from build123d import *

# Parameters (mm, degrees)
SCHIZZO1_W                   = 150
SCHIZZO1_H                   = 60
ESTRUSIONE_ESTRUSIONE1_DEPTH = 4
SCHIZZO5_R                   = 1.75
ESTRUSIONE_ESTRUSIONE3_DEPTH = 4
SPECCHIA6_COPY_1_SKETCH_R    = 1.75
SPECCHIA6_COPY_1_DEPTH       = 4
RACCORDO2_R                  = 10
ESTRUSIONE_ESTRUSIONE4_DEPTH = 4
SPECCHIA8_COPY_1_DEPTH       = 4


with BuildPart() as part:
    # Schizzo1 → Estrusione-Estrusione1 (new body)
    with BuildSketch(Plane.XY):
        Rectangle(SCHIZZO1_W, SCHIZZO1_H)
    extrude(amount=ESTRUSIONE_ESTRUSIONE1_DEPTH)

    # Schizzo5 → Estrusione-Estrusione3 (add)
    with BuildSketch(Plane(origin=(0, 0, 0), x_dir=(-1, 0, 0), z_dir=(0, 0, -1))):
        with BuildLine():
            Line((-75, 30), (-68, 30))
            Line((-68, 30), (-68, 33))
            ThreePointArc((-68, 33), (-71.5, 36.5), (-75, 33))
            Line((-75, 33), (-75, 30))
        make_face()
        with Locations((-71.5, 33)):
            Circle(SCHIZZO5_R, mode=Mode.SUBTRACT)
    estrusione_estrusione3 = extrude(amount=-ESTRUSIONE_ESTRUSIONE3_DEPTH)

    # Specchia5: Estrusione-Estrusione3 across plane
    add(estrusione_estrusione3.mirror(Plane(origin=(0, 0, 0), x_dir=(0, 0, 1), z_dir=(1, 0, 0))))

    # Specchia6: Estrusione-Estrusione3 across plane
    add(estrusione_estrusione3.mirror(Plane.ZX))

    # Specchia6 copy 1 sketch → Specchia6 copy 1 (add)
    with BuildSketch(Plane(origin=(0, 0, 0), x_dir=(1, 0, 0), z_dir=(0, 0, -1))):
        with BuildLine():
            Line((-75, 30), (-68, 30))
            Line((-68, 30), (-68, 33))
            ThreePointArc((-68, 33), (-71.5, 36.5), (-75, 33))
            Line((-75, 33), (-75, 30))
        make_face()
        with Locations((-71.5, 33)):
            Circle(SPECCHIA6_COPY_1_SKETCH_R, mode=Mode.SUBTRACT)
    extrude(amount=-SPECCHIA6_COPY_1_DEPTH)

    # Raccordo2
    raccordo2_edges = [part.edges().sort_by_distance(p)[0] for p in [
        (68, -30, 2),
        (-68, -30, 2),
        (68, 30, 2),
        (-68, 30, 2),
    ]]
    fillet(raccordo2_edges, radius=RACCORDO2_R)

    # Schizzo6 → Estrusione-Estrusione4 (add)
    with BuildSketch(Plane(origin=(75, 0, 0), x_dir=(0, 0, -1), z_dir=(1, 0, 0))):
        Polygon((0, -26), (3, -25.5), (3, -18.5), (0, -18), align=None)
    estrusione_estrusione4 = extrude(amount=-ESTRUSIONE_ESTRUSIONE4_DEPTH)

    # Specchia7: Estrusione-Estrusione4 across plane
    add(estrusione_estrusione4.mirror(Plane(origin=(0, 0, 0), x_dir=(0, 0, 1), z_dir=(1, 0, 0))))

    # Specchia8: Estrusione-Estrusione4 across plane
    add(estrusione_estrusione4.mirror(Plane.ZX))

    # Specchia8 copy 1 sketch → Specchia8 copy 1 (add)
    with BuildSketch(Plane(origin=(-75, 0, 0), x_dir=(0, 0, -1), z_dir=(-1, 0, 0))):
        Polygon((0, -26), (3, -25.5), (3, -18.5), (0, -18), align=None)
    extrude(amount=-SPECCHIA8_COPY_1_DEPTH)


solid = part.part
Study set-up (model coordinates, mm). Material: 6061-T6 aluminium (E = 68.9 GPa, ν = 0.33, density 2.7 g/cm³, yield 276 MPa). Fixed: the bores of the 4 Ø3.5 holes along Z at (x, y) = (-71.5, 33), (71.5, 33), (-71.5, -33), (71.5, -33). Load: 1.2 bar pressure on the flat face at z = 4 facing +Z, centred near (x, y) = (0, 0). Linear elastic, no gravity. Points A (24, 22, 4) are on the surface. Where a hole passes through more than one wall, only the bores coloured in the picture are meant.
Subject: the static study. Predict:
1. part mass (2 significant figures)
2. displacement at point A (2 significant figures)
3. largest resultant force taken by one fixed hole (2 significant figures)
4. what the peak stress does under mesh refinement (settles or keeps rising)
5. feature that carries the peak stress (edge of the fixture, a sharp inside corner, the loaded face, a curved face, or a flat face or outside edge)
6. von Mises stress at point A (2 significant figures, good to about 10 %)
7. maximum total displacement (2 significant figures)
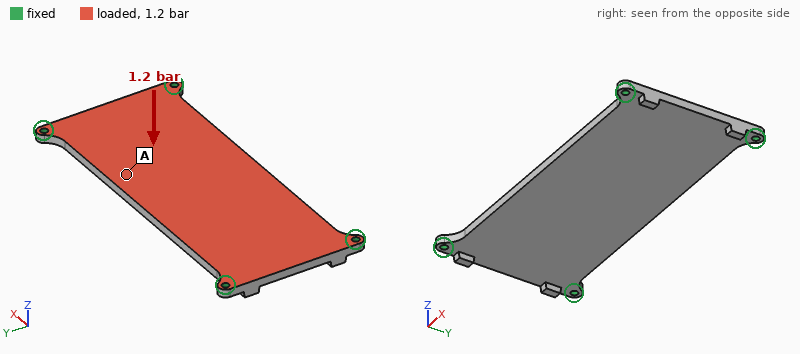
100 g
0.51 mm
280 N
keeps rising
edge of the fixture
41 MPa
0.63 mm
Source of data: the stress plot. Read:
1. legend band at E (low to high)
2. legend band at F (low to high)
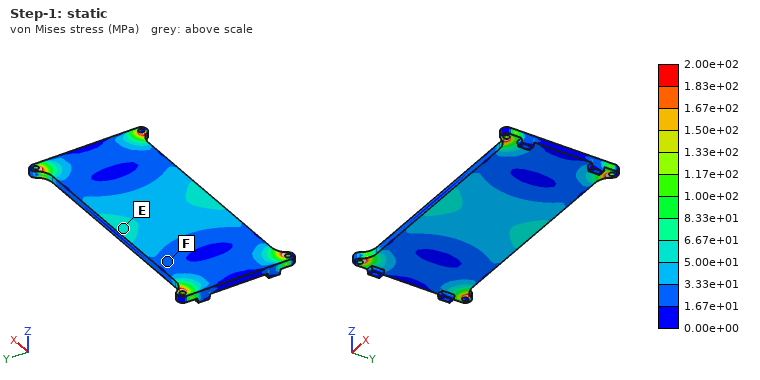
5.00e+01 to 6.67e+01 MPa
1.67e+01 to 3.33e+01 MPa
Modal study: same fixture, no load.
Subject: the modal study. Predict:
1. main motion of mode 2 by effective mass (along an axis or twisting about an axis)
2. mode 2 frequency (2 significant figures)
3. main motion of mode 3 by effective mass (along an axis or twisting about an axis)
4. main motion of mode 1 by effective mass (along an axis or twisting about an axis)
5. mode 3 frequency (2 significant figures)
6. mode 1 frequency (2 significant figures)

twisting about X
1800 Hz
twisting about Y
along Z
2200 Hz
770 Hz
